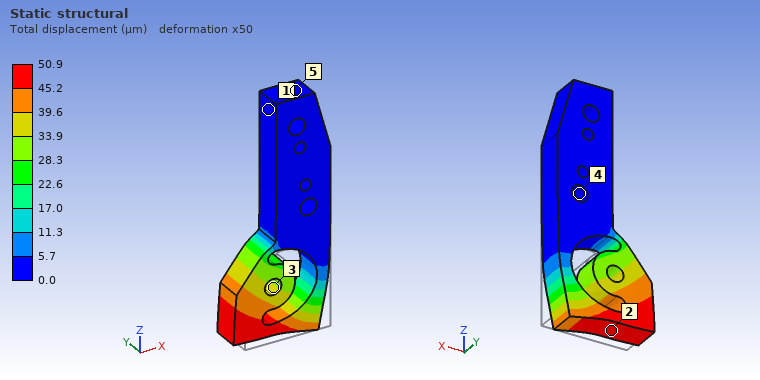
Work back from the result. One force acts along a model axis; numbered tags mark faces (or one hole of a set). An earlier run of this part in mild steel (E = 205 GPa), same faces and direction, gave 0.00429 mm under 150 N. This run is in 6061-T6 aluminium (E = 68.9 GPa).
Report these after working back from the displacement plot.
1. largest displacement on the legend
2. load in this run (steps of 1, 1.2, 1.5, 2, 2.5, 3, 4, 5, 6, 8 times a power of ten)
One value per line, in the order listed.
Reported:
50.9 µm
600 N
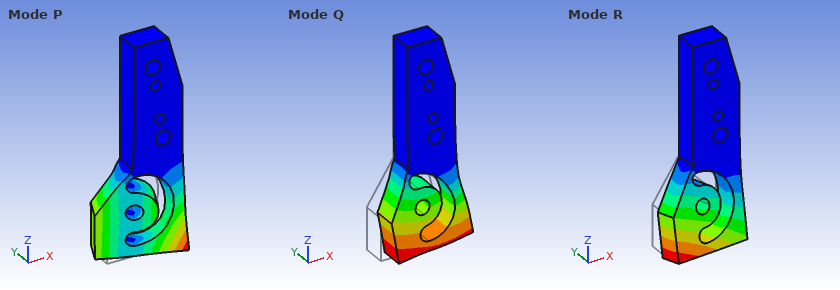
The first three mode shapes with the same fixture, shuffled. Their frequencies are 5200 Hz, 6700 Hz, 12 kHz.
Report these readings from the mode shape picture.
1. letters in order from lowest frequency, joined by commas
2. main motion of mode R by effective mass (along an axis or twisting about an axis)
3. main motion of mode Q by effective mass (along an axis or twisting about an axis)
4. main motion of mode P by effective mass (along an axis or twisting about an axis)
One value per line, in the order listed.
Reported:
R, Q, P
along Y
along X
twisting about Z
